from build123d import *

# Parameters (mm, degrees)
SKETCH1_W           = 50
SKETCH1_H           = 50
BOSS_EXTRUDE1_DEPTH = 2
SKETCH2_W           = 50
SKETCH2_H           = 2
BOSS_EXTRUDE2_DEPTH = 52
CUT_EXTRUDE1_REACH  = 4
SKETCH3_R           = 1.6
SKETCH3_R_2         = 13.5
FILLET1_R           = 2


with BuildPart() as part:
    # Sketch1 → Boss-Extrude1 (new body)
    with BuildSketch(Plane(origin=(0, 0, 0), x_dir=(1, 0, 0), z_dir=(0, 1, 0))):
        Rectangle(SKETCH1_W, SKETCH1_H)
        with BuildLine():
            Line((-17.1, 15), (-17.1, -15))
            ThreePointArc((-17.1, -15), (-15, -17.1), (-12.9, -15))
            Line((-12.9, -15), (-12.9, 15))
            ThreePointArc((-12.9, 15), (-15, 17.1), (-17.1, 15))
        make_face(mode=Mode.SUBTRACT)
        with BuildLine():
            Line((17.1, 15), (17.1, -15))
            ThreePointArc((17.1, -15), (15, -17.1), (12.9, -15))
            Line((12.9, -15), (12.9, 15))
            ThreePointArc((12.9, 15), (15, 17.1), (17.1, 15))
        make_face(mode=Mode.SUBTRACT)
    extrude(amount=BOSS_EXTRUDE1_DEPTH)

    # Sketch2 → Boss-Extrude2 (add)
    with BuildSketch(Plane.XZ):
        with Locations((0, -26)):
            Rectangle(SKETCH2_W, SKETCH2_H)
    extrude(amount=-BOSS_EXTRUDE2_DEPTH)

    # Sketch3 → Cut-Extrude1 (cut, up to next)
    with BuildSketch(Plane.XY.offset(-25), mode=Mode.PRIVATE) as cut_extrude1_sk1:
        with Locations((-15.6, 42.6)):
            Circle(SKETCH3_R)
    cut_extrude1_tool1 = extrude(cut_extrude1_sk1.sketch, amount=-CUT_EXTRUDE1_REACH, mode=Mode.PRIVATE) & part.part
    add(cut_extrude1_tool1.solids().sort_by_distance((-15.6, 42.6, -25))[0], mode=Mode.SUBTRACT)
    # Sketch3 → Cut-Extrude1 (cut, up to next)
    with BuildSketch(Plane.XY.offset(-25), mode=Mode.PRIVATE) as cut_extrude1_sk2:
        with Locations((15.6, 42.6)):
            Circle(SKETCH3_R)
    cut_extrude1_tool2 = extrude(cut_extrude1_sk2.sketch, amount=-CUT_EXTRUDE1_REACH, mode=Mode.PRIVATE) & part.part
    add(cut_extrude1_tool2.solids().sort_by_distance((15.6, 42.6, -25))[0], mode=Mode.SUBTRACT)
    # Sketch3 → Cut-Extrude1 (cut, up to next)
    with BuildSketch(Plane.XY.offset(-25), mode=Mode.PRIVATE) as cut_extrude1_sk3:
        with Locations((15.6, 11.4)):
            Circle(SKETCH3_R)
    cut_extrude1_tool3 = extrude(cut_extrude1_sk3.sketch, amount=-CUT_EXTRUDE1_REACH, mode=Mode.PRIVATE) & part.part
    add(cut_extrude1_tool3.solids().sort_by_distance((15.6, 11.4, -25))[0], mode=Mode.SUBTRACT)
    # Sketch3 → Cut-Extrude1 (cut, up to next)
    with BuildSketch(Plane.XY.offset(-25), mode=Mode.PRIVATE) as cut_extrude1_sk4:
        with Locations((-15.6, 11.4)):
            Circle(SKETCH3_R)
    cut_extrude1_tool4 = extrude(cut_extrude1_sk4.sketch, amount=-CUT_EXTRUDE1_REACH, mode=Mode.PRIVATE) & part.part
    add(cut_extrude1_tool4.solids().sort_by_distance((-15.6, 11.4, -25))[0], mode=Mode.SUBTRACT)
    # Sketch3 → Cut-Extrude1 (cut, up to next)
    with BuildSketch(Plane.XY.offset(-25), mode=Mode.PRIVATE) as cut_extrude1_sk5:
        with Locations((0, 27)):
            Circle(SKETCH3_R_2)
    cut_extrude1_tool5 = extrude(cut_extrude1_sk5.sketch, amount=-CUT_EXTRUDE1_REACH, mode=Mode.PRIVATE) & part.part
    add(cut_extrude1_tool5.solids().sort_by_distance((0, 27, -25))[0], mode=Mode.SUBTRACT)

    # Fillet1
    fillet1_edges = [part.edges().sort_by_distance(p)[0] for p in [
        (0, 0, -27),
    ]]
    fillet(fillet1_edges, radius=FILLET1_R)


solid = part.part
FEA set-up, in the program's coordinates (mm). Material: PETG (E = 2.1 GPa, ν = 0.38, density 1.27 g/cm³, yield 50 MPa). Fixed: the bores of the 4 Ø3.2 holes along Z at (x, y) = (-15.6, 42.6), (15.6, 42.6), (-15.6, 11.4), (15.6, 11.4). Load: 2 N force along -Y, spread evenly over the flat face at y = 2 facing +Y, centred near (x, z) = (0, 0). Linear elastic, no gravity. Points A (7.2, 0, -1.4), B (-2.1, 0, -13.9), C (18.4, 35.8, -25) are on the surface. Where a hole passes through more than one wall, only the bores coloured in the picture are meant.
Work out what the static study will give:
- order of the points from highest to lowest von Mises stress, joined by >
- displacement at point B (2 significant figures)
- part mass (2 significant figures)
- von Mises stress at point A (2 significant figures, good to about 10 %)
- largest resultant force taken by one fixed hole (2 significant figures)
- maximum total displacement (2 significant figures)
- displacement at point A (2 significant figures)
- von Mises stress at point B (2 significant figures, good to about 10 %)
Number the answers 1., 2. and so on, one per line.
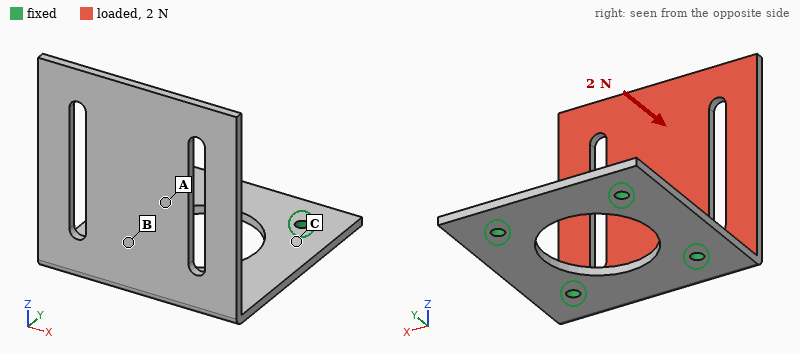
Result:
1. B > A > C
2. 0.15 mm
3. 11 g
4. 0.50 MPa
5. 1.1 N
6. 0.88 mm
7. 0.35 mm
8. 0.92 MPa
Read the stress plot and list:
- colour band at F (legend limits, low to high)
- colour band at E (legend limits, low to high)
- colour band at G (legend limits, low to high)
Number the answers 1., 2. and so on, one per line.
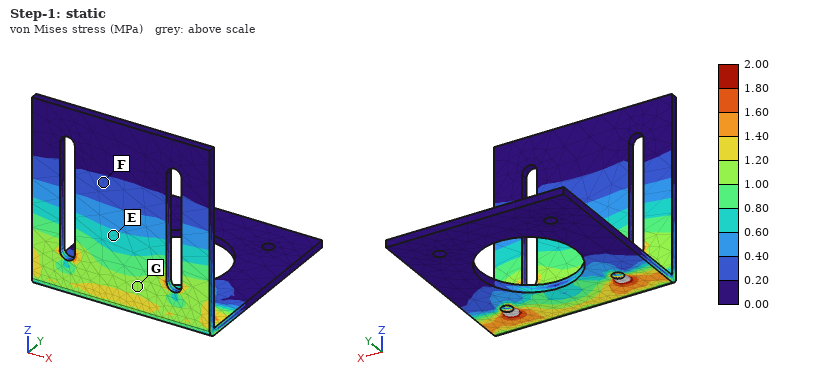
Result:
1. 0.20 to 0.40 MPa
2. 0.60 to 0.80 MPa
3. 1.00 to 1.20 MPa
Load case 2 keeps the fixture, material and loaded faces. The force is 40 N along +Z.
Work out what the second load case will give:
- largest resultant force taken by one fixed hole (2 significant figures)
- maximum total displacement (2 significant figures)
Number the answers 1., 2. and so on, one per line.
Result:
1. 21 N
2. 0.93 mm
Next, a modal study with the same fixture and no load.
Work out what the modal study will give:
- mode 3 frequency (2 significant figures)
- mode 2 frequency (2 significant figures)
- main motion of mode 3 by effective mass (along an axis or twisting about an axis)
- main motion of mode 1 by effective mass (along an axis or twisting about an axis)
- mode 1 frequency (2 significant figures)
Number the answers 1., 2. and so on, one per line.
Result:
1. 540 Hz
2. 330 Hz
3. along X
4. along Y
5. 120 Hz
